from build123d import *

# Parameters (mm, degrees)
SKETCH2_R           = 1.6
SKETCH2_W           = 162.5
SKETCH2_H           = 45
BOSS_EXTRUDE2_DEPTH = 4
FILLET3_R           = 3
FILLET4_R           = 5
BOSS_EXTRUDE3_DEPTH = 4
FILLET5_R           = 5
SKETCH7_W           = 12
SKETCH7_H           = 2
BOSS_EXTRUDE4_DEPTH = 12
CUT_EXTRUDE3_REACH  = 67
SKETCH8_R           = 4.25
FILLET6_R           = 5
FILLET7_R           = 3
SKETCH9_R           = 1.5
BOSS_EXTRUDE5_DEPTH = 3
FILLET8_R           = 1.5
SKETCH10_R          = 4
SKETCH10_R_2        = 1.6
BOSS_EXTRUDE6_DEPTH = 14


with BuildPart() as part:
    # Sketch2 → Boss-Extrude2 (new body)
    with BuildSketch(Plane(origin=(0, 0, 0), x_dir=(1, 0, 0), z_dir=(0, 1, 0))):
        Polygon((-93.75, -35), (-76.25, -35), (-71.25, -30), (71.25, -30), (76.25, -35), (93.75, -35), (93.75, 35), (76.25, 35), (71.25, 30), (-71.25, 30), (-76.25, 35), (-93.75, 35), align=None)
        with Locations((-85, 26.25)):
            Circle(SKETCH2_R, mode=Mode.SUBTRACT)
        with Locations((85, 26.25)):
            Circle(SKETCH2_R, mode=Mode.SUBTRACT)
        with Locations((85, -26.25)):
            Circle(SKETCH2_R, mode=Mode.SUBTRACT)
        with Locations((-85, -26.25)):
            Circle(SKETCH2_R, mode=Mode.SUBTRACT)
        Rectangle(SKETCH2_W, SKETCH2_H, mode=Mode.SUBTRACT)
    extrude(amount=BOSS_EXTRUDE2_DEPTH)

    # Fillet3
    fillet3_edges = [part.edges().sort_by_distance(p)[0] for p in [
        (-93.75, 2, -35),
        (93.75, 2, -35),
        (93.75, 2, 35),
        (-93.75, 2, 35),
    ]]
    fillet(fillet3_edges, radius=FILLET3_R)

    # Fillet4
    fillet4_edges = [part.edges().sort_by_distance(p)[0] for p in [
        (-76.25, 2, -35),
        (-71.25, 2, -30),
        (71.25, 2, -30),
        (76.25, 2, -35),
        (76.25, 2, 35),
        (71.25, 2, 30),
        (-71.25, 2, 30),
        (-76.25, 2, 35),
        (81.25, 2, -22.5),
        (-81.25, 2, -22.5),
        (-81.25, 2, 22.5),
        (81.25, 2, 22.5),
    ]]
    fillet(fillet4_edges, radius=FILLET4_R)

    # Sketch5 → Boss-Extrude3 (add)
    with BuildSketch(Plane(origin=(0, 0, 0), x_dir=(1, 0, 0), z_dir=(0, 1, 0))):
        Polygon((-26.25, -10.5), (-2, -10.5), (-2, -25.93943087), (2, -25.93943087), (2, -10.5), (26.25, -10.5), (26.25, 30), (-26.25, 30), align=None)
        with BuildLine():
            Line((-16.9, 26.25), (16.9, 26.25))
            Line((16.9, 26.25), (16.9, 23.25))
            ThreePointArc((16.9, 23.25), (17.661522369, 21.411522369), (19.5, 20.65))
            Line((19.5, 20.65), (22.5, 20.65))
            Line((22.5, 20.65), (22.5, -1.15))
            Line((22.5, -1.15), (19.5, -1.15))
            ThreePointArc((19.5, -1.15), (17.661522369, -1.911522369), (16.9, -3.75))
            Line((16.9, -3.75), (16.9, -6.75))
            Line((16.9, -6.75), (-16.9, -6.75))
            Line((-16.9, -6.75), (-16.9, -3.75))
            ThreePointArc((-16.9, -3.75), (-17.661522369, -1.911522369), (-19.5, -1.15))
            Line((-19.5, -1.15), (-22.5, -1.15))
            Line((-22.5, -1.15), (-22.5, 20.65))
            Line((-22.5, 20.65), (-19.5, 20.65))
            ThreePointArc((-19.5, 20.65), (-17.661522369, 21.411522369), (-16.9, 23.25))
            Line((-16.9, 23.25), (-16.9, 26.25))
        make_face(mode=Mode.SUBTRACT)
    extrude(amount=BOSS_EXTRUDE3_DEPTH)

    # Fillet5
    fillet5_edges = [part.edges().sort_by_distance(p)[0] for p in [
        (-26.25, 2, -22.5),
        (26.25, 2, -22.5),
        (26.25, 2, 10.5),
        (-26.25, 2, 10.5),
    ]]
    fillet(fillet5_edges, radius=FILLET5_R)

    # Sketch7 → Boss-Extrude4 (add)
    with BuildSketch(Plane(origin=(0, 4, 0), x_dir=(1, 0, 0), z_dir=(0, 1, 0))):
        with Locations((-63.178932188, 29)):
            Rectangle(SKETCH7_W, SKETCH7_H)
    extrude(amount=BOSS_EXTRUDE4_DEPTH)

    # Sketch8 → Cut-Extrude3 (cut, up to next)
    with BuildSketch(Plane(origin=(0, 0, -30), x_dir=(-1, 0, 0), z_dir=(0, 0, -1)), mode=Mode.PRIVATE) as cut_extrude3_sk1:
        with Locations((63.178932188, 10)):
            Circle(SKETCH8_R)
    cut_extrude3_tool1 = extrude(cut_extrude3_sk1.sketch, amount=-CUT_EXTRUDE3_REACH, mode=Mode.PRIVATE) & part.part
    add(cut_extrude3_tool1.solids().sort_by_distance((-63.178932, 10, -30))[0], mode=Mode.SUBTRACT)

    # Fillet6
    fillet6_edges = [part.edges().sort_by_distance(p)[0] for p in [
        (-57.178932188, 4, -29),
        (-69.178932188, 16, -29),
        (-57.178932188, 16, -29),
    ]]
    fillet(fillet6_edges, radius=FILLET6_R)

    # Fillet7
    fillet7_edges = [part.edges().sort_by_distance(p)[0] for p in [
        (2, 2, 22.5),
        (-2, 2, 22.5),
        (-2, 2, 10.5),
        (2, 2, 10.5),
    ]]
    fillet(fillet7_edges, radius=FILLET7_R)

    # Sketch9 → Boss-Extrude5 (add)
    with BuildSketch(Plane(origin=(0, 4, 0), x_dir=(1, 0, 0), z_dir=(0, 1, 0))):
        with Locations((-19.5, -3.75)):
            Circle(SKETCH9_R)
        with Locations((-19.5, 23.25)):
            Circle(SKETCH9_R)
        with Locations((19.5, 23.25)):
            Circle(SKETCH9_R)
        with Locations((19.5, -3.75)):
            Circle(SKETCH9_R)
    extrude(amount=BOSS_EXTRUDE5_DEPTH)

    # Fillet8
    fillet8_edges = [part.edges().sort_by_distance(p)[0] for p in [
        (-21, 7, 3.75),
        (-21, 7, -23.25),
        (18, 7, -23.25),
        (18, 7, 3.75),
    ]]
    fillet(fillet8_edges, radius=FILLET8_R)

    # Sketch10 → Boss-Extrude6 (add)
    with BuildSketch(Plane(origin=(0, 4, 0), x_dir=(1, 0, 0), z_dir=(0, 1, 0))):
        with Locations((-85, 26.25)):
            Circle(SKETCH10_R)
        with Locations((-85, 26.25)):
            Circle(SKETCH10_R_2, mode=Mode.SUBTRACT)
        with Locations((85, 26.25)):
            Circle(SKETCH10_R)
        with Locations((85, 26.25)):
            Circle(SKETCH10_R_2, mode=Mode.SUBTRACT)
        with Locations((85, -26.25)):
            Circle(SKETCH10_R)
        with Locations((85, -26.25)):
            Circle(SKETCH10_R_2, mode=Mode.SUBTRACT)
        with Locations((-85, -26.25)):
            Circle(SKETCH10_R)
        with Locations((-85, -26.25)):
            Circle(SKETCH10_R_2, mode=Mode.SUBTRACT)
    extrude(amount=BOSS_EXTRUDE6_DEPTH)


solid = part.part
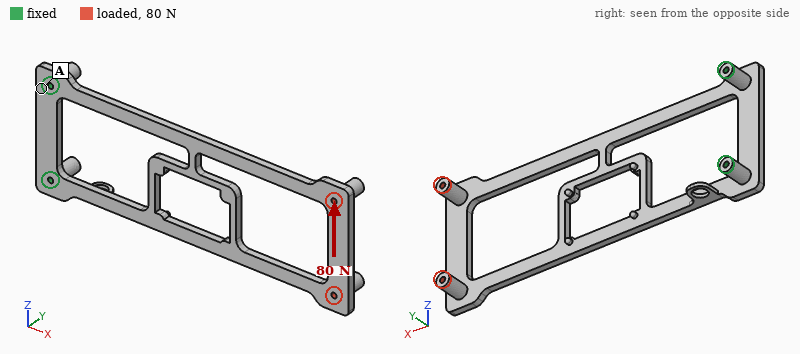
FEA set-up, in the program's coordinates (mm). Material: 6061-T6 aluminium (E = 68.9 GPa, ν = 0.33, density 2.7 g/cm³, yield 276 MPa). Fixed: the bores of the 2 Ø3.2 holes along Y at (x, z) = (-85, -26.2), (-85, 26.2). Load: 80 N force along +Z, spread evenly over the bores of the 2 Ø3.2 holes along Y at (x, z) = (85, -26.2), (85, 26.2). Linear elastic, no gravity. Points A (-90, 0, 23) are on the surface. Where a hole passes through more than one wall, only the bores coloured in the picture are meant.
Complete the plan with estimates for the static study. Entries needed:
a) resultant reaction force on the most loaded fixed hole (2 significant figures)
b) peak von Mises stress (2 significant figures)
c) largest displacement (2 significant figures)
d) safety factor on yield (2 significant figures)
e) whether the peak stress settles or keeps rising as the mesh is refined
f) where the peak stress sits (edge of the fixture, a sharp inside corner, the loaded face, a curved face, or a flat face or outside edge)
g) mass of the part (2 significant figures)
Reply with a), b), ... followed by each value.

a) 230 N
b) 82 MPa
c) 0.67 mm
d) 3.4
e) settles
f) a curved face
g) 60 g
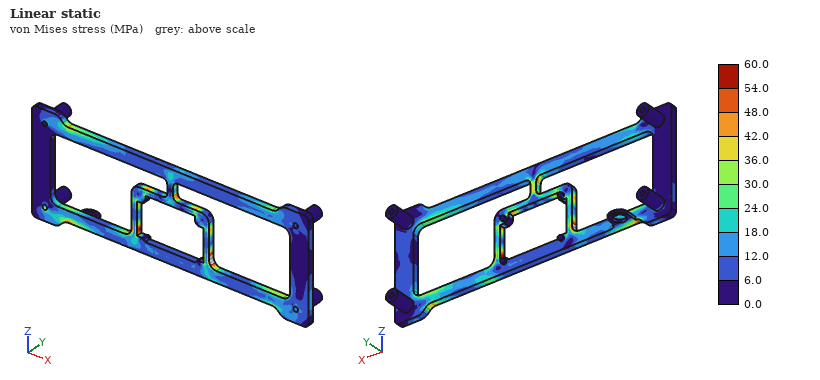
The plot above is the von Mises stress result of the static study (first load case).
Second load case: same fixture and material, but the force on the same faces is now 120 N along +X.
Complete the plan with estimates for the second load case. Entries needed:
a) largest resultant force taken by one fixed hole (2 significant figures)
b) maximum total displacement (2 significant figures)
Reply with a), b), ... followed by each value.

a) 60 N
b) 2.1 mm
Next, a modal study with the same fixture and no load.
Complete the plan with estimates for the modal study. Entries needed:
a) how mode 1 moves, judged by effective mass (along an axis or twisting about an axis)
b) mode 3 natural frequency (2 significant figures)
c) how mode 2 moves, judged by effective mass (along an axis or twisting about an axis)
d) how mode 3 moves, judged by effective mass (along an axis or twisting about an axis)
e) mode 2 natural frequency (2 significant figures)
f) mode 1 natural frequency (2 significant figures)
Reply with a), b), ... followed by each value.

a) along Y
b) 470 Hz
c) twisting about X
d) along Z
e) 310 Hz
f) 71 Hz
